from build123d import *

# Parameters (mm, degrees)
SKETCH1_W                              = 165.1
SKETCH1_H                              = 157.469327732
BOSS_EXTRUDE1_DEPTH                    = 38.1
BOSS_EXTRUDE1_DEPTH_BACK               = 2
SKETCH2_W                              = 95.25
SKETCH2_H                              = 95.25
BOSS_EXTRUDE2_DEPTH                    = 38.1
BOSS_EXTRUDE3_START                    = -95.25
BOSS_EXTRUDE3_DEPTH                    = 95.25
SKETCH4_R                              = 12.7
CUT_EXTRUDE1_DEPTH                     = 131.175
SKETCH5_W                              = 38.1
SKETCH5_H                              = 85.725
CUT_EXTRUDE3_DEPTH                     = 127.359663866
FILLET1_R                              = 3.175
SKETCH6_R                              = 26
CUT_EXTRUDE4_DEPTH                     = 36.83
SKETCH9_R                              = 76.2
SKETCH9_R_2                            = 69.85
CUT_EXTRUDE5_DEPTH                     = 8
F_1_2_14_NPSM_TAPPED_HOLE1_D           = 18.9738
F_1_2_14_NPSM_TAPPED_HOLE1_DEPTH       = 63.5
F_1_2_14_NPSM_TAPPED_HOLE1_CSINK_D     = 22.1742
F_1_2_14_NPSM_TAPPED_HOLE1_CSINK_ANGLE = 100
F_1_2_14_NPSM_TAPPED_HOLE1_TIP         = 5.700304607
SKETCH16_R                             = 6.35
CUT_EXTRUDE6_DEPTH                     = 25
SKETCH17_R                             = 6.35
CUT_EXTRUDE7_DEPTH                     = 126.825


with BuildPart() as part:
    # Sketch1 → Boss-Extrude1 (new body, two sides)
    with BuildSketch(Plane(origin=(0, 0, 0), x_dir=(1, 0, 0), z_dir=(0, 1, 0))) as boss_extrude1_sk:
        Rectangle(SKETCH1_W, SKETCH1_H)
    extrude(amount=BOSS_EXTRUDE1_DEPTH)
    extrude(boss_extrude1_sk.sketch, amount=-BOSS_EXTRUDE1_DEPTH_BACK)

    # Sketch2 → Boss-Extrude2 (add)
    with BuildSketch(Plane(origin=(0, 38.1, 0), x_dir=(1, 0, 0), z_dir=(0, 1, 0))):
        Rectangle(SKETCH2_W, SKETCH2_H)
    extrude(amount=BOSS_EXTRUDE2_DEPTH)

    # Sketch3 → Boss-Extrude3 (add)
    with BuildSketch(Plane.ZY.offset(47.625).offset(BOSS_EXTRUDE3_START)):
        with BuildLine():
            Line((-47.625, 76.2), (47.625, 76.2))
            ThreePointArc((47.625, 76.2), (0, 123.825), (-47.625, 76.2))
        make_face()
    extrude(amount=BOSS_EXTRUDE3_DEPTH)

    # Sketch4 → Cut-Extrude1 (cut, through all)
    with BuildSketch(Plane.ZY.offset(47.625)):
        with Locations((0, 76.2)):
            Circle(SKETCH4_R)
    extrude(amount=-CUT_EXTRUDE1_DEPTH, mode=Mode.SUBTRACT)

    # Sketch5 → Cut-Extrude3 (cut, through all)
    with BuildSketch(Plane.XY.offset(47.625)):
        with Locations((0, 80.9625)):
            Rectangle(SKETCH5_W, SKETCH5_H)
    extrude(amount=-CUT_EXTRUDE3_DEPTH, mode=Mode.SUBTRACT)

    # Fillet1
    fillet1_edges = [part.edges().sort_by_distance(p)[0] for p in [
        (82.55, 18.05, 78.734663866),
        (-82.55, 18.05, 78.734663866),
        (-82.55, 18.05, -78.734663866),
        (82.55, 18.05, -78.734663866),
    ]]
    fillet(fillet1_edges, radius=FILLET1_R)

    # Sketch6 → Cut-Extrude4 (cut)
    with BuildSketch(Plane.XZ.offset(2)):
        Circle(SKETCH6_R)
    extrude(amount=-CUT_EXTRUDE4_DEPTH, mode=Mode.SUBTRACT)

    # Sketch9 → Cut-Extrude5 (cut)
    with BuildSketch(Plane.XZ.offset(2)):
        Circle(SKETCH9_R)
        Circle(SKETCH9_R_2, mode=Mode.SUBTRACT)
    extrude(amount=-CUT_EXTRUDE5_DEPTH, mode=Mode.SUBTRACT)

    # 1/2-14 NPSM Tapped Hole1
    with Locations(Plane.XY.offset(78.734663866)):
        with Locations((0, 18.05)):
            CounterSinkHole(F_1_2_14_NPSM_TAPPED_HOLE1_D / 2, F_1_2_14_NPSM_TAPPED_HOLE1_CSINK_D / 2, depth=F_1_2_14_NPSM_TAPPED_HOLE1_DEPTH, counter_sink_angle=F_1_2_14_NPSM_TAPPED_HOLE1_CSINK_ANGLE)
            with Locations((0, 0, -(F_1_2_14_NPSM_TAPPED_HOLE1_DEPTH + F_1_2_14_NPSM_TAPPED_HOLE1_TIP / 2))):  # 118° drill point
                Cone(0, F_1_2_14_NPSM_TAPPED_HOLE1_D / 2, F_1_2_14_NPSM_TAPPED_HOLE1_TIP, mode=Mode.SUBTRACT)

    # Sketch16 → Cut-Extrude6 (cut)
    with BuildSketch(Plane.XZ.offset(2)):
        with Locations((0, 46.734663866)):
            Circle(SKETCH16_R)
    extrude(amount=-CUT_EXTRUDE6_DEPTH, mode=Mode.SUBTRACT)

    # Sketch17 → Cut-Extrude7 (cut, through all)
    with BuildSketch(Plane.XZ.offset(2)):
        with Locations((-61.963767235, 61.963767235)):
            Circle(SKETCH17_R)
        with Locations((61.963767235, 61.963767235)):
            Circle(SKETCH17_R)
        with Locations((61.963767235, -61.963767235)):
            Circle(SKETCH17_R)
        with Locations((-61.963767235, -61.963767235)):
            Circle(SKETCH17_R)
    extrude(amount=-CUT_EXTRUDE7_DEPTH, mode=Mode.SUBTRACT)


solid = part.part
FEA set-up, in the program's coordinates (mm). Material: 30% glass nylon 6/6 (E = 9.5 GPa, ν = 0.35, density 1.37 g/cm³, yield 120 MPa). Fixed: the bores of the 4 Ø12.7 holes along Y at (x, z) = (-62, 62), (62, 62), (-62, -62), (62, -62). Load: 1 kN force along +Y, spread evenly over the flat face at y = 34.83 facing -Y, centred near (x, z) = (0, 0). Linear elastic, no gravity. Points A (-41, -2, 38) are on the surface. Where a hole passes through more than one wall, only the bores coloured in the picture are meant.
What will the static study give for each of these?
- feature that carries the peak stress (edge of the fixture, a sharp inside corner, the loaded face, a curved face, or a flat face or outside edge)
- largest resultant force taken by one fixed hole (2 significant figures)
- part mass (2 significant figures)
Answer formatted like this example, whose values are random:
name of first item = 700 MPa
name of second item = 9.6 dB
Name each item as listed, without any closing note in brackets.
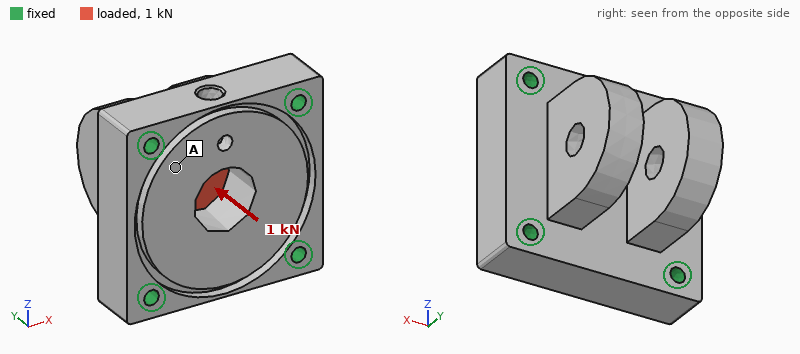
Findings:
feature that carries the peak stress = a flat face or outside edge
largest resultant force taken by one fixed hole = 260 N
part mass = 1.8 kg
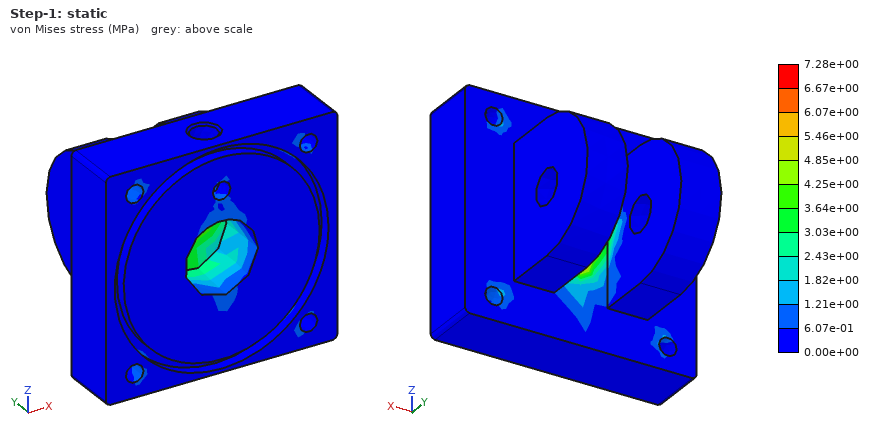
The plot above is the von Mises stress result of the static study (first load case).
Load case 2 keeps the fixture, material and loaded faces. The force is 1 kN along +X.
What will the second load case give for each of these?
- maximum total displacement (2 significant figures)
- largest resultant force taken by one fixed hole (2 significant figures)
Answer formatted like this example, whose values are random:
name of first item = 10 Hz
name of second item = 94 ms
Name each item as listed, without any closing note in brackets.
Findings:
maximum total displacement = 5.8 µm
largest resultant force taken by one fixed hole = 290 N
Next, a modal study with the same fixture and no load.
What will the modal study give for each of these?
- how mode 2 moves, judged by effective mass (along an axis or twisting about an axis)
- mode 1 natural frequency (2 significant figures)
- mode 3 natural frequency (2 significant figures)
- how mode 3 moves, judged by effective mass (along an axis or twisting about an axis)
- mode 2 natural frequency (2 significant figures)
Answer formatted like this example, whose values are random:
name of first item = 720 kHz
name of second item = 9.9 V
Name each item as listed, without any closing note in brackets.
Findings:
how mode 2 moves, judged by effective mass = along X
mode 1 natural frequency = 1300 Hz
mode 3 natural frequency = 2400 Hz
how mode 3 moves, judged by effective mass = along Z
mode 2 natural frequency = 1400 Hz
